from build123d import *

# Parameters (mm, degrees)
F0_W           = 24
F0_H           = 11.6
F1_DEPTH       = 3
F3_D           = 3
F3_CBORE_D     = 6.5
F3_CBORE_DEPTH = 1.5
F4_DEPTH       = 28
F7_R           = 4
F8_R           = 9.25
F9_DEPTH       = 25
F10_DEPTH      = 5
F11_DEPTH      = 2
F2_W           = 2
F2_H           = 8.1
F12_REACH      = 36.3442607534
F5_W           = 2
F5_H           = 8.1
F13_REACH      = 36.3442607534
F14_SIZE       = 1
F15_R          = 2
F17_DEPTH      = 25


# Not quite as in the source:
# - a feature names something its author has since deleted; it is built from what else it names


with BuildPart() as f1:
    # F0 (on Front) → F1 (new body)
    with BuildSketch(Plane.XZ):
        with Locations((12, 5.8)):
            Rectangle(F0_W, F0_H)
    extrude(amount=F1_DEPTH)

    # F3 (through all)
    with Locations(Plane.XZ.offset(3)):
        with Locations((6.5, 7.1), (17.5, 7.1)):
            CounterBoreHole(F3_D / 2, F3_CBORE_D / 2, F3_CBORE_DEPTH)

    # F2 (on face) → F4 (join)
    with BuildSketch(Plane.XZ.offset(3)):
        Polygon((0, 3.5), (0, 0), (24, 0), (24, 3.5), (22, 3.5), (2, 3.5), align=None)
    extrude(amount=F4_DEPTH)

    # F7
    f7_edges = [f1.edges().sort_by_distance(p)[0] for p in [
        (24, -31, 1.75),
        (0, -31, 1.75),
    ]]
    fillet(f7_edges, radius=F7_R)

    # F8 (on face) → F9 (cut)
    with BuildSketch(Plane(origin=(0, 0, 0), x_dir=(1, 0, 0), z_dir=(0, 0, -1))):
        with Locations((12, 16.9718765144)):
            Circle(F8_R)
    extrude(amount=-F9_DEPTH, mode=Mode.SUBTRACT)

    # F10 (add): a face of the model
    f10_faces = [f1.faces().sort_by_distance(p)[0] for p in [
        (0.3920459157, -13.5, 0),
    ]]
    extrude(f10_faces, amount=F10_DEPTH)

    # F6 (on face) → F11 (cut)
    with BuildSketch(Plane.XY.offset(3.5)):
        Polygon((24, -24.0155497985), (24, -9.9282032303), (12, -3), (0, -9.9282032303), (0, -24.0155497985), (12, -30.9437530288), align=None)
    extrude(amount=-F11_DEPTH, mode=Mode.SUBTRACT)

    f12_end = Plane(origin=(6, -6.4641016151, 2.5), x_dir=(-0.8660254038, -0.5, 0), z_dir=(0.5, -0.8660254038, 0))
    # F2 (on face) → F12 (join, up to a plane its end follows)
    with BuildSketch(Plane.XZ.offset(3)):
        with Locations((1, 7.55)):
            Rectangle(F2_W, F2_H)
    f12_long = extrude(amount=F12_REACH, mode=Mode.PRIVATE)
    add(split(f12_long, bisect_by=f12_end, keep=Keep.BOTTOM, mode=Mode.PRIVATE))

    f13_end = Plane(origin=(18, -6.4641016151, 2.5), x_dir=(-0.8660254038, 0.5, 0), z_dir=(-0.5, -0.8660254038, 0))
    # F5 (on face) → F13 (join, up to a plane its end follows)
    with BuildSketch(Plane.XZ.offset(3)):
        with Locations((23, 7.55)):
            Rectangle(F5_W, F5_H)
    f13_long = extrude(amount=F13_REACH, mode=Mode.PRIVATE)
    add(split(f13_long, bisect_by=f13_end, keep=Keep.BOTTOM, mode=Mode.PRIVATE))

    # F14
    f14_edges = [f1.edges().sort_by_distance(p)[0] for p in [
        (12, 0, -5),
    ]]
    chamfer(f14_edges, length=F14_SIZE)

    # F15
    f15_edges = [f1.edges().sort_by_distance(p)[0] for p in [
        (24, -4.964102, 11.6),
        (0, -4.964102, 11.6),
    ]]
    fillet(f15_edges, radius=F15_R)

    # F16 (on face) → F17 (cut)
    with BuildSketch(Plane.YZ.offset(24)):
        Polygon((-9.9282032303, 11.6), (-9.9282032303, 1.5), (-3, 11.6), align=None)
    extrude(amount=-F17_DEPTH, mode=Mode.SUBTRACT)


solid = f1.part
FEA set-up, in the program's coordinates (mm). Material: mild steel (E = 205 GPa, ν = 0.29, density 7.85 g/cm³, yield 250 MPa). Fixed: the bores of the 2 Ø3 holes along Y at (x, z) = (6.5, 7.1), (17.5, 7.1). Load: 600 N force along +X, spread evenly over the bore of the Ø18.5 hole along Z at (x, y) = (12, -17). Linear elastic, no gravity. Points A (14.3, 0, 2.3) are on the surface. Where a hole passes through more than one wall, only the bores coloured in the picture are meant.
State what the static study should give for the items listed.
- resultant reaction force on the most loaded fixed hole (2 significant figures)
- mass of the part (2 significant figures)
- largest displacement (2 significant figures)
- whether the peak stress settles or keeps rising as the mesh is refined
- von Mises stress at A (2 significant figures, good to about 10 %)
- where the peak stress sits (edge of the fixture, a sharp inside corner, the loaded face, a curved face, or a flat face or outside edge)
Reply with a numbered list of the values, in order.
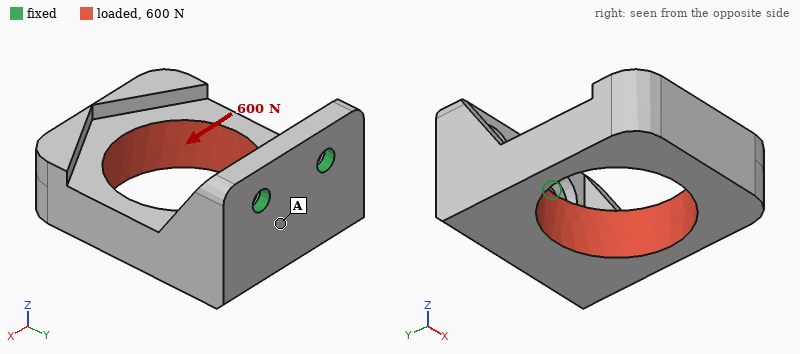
1. 890 N
2. 32 g
3. 52 µm
4. keeps rising
5. 33 MPa
6. edge of the fixture
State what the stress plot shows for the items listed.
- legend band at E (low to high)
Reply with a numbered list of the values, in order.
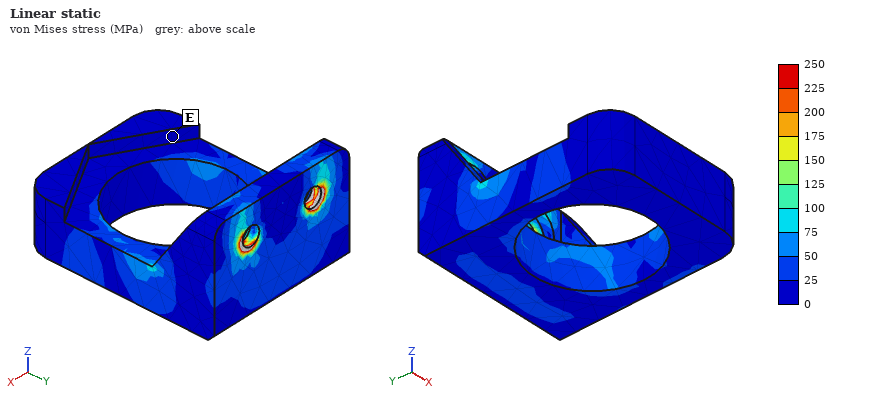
1. 0 to 25 MPa
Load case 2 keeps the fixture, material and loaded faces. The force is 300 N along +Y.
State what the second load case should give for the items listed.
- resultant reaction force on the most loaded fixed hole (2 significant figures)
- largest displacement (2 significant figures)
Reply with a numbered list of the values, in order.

1. 150 N
2. 49 µm
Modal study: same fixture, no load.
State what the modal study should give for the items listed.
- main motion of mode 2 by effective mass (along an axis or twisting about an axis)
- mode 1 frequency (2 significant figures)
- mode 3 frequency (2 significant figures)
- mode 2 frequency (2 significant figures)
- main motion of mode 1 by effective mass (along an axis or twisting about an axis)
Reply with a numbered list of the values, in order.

1. along X
2. 1900 Hz
3. 9300 Hz
4. 4000 Hz
5. along Z
